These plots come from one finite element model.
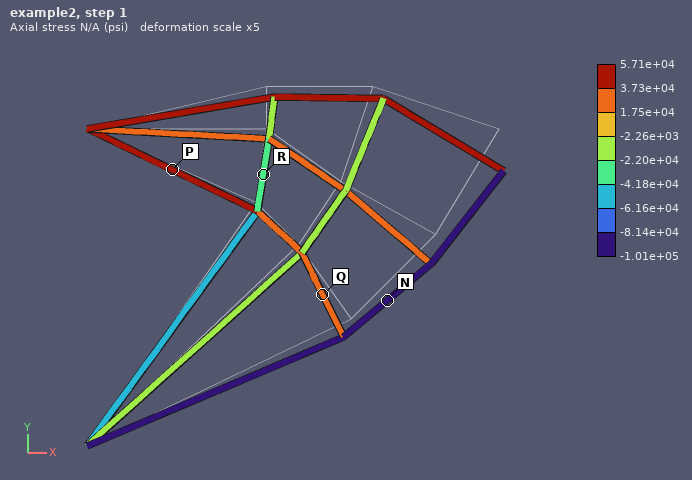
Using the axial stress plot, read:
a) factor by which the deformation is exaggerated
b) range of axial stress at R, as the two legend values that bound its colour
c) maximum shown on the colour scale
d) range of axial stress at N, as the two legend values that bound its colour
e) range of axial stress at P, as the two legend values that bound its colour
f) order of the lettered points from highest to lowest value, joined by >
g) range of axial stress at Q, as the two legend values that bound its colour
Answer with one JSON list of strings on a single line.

["5", "-4.18e+04 to -2.20e+04 psi", "5.71e+04 psi", "-1.01e+05 to -8.14e+04 psi", "3.73e+04 to 5.71e+04 psi", "P > Q > R > N", "1.75e+04 to 3.73e+04 psi"]
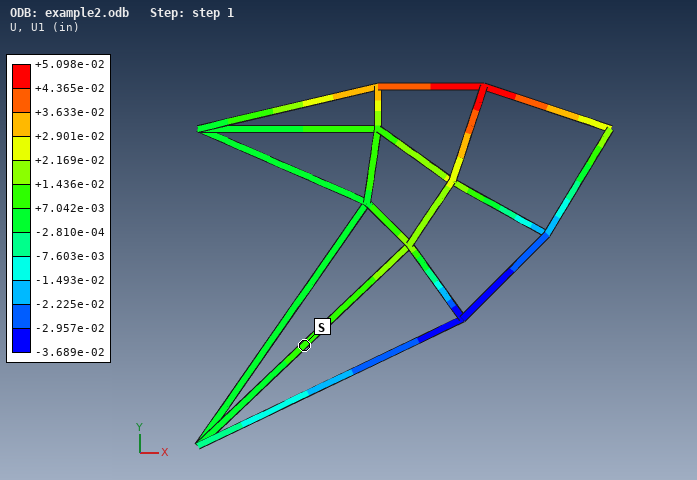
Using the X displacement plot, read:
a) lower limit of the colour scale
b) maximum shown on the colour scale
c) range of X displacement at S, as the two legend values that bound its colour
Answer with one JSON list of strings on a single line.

["-3.689e-02 in", "+5.098e-02 in", "+7.042e-03 to +1.436e-02 in"]
